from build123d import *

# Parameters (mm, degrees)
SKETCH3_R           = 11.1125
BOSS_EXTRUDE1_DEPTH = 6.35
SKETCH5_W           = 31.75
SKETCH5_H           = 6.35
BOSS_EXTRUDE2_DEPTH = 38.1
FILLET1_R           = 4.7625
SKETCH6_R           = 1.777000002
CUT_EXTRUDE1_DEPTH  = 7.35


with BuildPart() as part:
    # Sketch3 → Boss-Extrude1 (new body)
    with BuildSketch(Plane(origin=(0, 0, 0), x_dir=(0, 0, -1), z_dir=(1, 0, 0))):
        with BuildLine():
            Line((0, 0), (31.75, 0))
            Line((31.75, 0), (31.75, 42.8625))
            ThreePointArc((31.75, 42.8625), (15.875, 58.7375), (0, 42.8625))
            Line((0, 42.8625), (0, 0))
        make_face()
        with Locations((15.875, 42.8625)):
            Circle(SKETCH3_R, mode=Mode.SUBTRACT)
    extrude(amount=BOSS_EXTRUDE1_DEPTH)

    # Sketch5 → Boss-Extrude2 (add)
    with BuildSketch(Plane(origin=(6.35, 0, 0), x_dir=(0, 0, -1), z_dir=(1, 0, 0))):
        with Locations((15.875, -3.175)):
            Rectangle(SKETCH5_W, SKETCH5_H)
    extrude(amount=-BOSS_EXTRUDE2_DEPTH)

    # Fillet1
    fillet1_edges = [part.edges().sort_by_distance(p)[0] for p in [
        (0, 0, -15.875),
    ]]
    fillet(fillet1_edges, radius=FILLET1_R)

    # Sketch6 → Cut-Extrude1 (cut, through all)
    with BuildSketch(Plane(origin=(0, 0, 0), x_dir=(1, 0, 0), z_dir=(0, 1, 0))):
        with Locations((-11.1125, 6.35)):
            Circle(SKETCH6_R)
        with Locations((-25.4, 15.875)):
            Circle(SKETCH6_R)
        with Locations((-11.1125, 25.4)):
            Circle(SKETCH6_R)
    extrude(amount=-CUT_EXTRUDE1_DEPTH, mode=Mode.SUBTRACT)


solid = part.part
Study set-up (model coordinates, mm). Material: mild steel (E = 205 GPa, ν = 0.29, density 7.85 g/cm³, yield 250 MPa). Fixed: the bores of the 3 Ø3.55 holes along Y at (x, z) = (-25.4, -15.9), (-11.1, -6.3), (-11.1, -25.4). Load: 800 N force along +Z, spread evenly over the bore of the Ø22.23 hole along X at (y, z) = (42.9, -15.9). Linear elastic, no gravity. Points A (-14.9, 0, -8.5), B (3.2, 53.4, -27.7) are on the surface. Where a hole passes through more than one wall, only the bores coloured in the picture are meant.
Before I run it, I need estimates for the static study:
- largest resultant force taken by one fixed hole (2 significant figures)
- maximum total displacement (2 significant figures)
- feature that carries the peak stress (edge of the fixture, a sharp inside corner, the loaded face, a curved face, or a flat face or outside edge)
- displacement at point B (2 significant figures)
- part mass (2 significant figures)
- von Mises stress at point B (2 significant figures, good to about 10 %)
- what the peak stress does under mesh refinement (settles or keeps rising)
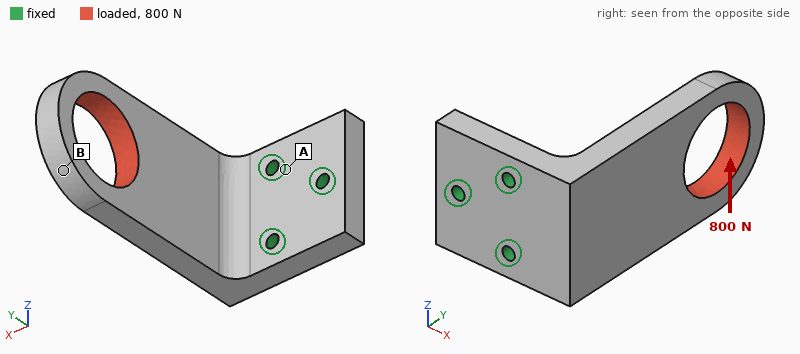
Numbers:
1.7 kN
79 µm
edge of the fixture
74 µm
130 g
27 MPa
keeps rising
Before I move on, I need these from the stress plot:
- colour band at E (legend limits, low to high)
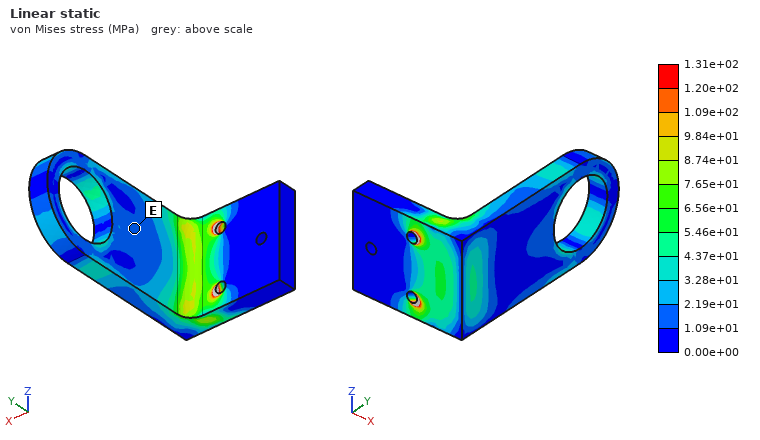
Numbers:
1.09e+01 to 2.19e+01 MPa
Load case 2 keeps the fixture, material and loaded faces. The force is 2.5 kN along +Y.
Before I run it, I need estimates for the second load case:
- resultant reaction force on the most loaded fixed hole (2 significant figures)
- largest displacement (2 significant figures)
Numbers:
1.5 kN
0.12 mm
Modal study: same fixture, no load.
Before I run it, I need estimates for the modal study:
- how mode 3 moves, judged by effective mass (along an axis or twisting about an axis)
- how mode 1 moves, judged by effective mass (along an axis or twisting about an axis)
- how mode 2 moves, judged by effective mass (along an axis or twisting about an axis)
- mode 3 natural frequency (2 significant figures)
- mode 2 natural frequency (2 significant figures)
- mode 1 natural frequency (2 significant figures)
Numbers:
along Y
along X
along Z
5900 Hz
3400 Hz
1500 Hz
